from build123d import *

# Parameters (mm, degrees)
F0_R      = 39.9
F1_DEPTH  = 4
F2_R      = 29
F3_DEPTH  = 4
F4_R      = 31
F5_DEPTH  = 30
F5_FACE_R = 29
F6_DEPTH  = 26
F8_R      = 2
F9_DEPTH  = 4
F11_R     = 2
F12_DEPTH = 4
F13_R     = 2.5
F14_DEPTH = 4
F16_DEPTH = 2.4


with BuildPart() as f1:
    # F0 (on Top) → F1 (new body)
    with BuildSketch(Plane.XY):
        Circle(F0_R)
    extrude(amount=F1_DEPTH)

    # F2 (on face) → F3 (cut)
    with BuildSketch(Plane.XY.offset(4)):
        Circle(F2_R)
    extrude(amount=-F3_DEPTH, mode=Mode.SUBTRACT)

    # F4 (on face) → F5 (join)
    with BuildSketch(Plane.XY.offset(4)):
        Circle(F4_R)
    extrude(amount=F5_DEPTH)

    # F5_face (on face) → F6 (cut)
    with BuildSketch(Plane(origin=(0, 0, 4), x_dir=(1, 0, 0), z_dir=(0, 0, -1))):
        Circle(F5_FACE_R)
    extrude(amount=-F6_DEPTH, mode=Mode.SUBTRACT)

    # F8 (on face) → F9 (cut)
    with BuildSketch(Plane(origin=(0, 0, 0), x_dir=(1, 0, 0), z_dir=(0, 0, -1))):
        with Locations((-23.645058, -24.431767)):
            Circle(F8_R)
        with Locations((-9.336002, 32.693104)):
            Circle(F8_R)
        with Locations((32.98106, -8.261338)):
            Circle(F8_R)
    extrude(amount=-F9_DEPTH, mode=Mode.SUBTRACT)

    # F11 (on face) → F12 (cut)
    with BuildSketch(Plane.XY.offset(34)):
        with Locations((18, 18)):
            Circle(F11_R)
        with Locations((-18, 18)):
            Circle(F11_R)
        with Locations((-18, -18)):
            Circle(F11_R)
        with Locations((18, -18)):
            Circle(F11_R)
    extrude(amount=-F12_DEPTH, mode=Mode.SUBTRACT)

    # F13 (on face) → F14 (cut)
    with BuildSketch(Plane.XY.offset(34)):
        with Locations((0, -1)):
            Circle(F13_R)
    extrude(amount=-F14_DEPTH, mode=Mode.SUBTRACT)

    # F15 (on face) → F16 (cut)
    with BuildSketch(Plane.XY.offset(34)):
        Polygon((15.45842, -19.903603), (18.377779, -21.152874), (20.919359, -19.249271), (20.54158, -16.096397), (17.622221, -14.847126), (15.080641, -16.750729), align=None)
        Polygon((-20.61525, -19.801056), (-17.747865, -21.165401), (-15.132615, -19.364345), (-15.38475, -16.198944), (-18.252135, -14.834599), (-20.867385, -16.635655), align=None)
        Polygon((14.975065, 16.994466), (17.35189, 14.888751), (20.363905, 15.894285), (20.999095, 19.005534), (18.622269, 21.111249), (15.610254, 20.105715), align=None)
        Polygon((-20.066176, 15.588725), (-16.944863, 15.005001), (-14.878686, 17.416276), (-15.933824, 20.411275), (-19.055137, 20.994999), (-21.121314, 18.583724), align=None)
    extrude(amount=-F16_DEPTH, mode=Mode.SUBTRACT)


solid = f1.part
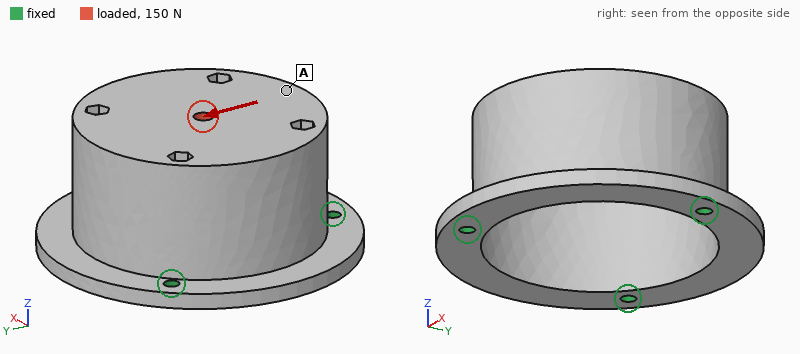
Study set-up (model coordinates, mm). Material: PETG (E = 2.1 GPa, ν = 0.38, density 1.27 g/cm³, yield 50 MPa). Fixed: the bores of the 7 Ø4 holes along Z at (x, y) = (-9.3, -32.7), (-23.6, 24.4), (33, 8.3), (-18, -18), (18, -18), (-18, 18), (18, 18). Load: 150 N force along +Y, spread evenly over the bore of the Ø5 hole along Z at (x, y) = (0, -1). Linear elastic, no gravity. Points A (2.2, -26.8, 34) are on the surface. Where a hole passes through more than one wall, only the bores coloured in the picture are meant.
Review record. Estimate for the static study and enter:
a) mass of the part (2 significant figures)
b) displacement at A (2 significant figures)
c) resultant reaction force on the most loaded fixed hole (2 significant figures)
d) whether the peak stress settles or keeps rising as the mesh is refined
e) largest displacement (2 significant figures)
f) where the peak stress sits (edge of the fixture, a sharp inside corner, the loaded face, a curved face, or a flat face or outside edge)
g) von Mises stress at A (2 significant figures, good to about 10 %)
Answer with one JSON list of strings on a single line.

["39 g", "8.2 µm", "39 N", "keeps rising", "17 µm", "edge of the fixture", "0.41 MPa"]
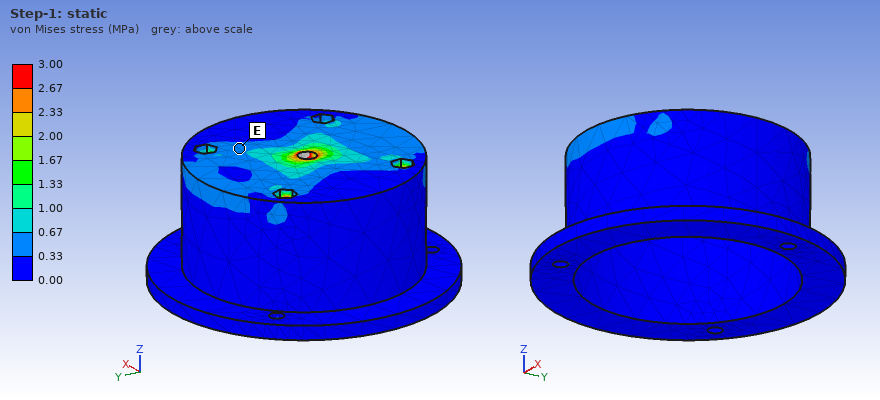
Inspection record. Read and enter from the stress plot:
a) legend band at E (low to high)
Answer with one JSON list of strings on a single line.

["0.33 to 0.67 MPa"]
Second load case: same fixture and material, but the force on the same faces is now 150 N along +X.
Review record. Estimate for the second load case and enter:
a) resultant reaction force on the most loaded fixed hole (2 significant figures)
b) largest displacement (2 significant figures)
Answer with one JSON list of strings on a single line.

["40 N", "17 µm"]
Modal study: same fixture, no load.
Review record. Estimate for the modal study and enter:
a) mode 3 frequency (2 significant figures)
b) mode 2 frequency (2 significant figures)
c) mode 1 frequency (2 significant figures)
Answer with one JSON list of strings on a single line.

["3000 Hz", "2900 Hz", "2600 Hz"]
